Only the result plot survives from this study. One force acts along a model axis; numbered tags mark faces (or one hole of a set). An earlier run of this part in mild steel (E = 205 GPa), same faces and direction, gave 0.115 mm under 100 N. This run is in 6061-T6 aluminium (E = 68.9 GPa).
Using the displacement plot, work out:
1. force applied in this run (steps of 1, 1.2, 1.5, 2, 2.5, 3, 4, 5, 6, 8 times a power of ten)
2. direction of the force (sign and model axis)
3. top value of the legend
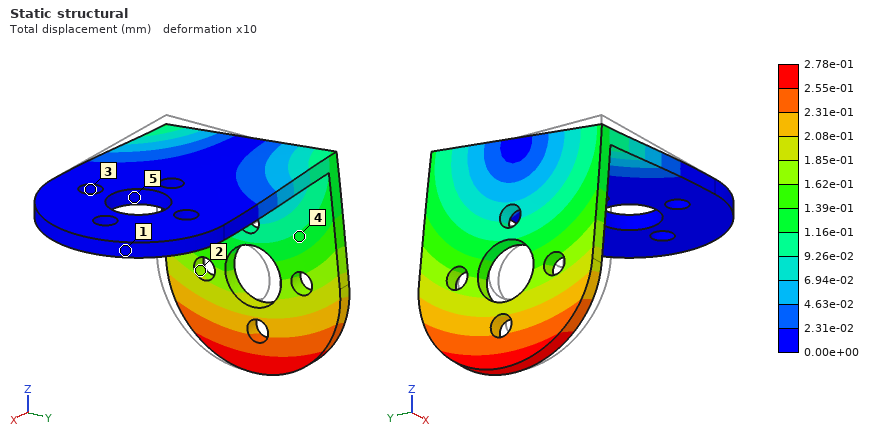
80 N
+Y
2.78e-01 mm
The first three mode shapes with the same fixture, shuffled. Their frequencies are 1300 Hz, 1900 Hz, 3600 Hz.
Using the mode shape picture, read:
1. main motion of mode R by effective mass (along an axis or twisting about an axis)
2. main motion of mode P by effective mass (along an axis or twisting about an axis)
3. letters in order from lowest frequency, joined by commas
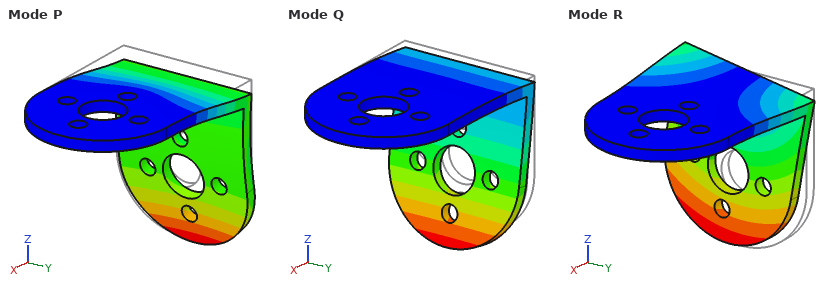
along Y
along Z
Q, R, P
